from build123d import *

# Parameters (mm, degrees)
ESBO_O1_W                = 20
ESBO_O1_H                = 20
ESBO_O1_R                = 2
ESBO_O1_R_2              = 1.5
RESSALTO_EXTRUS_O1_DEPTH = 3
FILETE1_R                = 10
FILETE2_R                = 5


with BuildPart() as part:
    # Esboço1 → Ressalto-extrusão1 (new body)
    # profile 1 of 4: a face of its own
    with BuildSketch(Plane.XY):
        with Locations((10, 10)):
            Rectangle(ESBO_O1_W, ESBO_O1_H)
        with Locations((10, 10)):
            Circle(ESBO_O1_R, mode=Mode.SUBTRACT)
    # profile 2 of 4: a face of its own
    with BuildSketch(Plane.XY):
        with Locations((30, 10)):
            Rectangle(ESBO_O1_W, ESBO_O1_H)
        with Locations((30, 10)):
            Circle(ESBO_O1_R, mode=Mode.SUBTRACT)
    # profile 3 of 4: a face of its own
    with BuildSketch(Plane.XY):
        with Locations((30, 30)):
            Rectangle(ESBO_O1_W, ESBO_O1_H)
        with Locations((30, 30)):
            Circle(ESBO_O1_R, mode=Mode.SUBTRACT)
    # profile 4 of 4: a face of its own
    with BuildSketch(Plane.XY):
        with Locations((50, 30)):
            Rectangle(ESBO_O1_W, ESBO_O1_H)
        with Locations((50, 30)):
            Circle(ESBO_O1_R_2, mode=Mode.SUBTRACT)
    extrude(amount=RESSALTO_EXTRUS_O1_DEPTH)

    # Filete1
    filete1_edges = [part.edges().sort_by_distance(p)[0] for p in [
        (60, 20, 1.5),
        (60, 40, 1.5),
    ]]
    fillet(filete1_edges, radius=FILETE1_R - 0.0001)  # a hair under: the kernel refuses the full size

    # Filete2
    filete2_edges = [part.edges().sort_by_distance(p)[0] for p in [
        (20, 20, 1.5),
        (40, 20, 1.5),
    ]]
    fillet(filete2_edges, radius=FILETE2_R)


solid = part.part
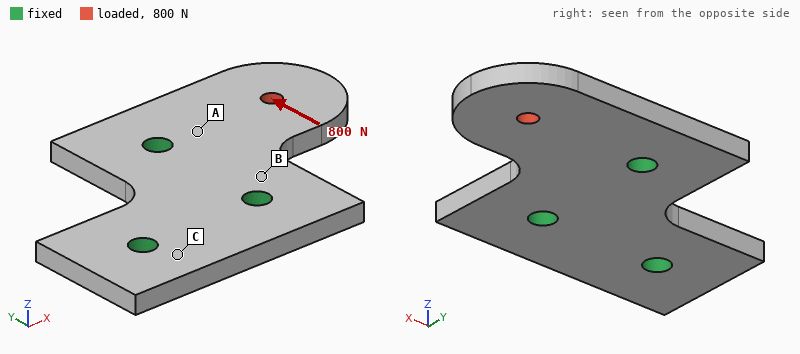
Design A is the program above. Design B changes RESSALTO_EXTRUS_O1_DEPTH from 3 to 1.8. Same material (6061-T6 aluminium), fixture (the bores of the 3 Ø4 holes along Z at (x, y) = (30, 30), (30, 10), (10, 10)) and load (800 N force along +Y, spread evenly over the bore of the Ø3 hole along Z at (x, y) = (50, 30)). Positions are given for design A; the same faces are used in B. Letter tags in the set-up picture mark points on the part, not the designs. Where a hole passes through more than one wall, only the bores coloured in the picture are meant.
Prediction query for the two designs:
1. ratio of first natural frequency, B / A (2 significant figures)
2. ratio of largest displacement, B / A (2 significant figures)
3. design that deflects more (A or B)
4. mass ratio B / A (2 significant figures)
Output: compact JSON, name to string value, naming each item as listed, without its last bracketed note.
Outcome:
{"ratio of first natural frequency, B / A": "0.62", "ratio of largest displacement, B / A": "1.7", "design that deflects more": "B", "mass ratio B / A": "0.60"}
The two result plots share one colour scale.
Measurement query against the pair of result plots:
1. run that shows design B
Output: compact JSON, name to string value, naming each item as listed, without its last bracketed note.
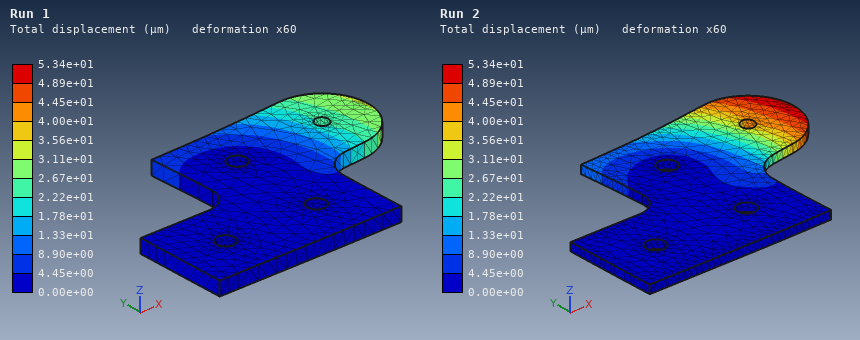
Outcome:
{"run that shows design B": "Run 2"}
